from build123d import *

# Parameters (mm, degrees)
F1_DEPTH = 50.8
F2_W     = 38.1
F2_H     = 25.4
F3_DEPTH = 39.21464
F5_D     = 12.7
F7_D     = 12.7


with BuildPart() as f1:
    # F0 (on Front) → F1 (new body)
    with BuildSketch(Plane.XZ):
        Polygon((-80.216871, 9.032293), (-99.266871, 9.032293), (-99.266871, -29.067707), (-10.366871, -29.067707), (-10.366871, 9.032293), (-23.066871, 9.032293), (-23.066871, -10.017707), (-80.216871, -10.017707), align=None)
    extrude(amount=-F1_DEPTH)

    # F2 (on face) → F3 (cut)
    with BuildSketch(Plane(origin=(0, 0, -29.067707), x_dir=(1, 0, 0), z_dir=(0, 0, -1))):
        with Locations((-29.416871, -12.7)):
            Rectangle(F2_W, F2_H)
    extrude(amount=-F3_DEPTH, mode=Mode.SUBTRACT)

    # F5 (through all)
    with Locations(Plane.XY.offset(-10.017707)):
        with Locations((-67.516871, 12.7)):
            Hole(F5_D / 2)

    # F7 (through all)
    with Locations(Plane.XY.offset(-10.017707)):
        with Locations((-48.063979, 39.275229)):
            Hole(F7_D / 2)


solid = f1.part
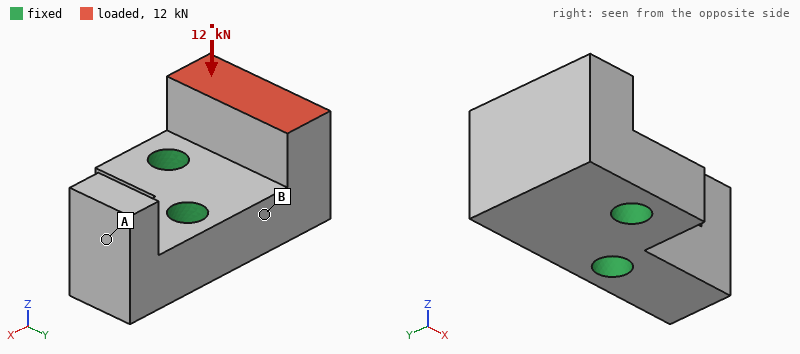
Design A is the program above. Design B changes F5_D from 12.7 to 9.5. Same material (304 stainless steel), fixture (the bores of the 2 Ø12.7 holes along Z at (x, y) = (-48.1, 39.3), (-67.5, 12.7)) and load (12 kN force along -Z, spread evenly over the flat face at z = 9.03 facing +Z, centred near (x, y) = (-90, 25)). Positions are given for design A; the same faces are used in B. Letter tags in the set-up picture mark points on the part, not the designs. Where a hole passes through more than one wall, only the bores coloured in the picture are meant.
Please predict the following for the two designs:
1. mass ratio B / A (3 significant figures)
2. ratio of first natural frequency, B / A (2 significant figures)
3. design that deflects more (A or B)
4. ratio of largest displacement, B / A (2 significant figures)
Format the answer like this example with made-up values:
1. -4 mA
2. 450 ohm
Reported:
1. 1.01
2. 0.93
3. B
4. 1.2
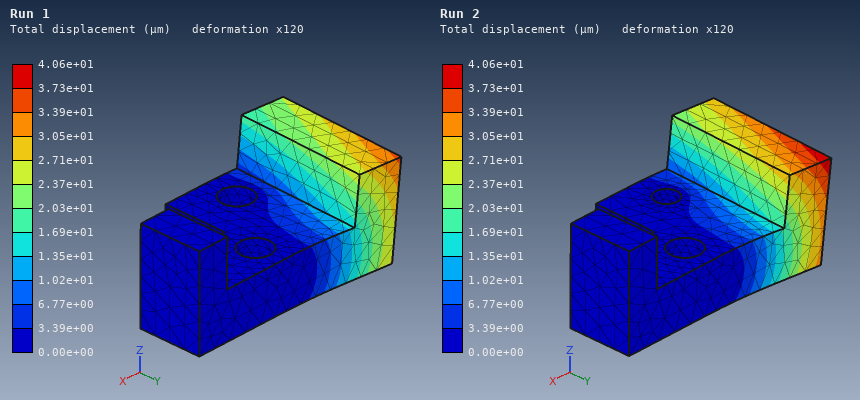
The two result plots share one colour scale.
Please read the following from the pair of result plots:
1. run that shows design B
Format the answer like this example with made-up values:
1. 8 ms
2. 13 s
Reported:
1. Run 2
